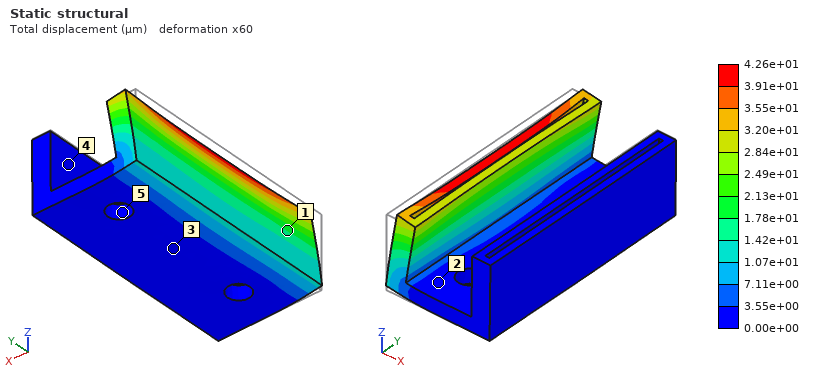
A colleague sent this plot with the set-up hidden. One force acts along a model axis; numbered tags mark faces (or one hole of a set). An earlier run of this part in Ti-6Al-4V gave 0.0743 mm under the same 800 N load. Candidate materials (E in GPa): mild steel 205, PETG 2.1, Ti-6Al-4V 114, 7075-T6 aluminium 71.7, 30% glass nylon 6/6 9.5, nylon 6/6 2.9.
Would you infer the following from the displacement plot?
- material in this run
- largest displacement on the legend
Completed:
mild steel
4.26e+01 µm
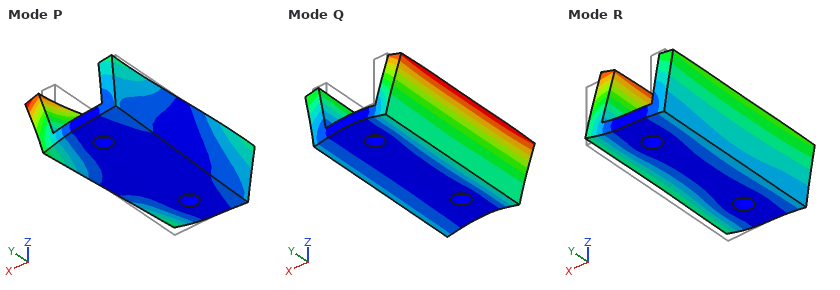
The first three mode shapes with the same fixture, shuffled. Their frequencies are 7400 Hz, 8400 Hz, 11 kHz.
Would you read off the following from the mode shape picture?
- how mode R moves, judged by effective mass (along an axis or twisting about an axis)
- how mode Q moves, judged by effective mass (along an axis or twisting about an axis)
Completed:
along X
along Z
